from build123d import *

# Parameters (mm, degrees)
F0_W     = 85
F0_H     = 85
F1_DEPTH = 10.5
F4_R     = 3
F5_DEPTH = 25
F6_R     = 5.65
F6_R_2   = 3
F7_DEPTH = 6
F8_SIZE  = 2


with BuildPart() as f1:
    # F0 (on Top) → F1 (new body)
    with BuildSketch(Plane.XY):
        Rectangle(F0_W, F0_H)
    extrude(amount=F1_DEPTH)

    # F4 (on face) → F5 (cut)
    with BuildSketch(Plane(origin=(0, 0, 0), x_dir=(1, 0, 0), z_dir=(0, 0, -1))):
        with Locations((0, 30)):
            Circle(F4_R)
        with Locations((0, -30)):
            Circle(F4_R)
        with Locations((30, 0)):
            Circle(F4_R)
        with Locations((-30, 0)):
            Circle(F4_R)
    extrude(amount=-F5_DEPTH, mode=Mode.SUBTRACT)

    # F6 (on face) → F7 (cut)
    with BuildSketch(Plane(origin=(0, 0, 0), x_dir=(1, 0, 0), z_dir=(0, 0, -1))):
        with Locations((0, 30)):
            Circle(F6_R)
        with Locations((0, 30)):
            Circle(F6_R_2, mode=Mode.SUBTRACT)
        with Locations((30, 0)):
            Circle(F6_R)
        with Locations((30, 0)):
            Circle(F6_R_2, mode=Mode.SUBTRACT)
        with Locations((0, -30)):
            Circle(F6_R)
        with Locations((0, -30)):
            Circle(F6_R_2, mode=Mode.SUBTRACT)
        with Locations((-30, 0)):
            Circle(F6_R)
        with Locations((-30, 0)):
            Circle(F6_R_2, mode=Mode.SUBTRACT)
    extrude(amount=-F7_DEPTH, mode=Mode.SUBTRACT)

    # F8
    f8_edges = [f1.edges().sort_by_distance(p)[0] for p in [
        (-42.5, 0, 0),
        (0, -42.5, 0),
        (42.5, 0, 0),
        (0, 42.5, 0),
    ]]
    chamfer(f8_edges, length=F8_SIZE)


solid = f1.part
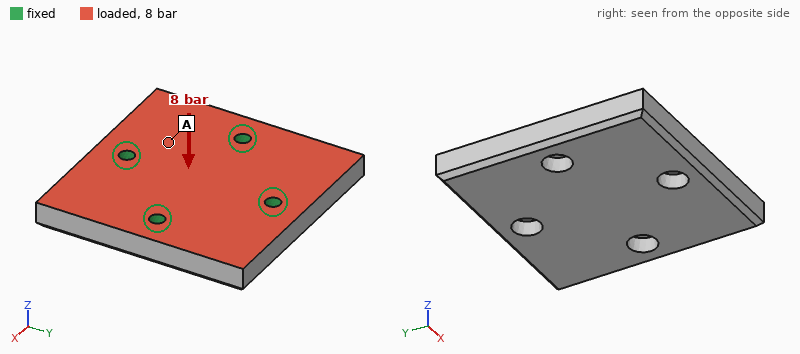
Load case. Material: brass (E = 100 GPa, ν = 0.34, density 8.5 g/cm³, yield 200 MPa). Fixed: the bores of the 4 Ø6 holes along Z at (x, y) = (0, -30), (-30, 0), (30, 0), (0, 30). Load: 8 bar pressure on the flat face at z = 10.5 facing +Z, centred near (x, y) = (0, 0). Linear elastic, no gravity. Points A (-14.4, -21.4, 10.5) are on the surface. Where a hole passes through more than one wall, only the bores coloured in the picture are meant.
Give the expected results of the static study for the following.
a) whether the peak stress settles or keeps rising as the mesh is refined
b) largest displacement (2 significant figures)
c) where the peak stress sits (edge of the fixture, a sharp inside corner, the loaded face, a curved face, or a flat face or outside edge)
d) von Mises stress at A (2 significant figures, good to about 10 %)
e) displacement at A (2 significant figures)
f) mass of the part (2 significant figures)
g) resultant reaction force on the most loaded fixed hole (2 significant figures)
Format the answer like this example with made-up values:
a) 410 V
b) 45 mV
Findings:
a) keeps rising
b) 17 µm
c) edge of the fixture
d) 7.7 MPa
e) 3.5 µm
f) 610 g
g) 1.4 kN
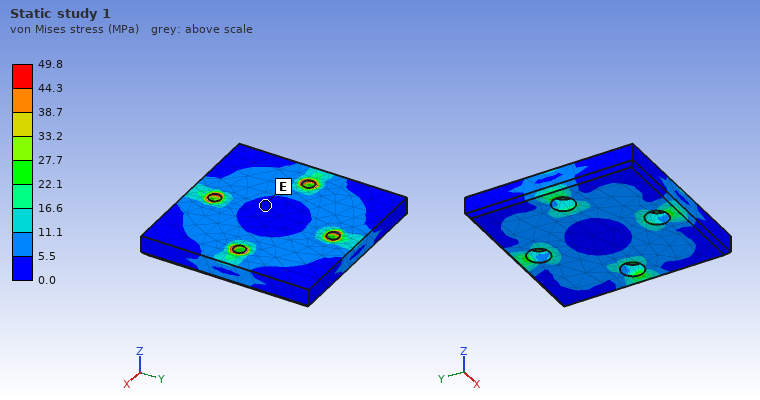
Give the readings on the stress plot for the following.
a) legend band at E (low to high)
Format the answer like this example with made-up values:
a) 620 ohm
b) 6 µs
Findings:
a) 0.0 to 5.5 MPa
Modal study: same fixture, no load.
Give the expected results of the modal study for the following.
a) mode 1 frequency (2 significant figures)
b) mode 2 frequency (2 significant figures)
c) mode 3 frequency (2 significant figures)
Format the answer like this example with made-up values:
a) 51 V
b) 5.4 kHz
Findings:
a) 4000 Hz
b) 4500 Hz
c) 4500 Hz
